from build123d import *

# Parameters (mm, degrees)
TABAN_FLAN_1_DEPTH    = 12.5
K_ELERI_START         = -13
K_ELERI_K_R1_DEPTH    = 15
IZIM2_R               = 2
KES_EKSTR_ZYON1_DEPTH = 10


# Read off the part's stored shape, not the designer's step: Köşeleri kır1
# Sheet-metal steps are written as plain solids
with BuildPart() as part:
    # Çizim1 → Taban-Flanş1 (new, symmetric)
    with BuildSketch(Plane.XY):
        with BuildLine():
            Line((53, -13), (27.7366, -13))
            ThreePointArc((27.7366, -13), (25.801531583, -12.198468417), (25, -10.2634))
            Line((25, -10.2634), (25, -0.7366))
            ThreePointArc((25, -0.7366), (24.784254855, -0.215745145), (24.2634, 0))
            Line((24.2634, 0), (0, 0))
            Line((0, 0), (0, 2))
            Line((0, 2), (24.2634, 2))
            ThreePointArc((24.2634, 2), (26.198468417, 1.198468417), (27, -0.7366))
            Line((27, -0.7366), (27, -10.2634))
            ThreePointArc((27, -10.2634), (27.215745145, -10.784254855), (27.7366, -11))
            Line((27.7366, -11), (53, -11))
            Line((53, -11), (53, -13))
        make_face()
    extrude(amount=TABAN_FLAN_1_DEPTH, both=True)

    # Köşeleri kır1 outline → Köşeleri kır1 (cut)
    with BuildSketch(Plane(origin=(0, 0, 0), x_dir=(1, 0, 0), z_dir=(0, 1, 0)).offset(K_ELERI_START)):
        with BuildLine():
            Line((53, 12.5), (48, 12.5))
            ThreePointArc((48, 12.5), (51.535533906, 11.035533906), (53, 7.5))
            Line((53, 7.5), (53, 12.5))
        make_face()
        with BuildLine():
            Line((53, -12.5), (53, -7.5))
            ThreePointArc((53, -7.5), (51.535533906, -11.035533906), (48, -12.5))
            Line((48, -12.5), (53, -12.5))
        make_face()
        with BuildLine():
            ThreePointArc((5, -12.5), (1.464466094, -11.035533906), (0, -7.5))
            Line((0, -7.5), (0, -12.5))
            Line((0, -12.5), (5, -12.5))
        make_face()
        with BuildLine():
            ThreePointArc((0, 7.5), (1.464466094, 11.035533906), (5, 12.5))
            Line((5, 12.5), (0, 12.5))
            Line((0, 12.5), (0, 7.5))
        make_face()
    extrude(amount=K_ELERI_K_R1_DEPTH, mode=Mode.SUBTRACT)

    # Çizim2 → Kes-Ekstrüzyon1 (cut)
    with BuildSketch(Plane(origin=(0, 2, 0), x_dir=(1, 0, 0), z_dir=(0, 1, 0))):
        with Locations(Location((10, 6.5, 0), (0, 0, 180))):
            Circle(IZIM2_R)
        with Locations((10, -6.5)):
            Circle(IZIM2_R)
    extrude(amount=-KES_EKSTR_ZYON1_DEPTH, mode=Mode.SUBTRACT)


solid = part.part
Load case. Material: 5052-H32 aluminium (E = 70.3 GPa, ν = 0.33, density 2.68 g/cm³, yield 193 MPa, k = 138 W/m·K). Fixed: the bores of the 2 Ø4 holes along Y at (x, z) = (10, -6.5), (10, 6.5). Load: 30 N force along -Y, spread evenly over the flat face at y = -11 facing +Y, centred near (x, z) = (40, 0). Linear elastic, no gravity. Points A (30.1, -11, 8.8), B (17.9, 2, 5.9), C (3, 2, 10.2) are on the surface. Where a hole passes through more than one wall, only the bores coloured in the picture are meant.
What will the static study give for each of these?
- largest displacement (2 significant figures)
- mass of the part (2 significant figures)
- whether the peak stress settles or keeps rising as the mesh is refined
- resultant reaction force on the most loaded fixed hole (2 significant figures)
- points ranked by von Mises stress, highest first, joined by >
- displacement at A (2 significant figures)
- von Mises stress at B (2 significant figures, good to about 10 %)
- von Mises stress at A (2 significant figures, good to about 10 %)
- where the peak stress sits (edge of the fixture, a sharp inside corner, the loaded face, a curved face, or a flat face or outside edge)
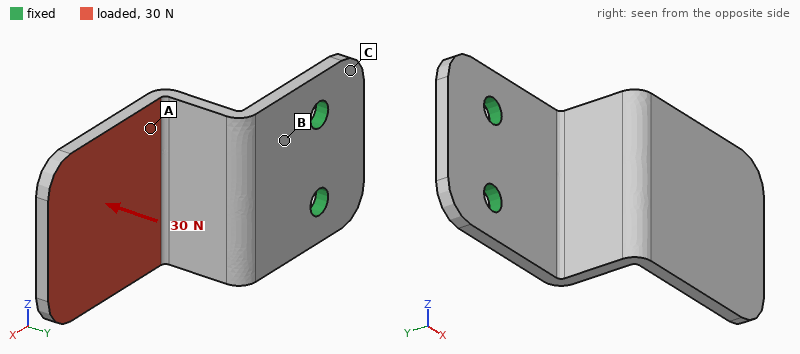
0.46 mm
8.4 g
keeps rising
15 N
B > A > C
0.16 mm
35 MPa
17 MPa
edge of the fixture
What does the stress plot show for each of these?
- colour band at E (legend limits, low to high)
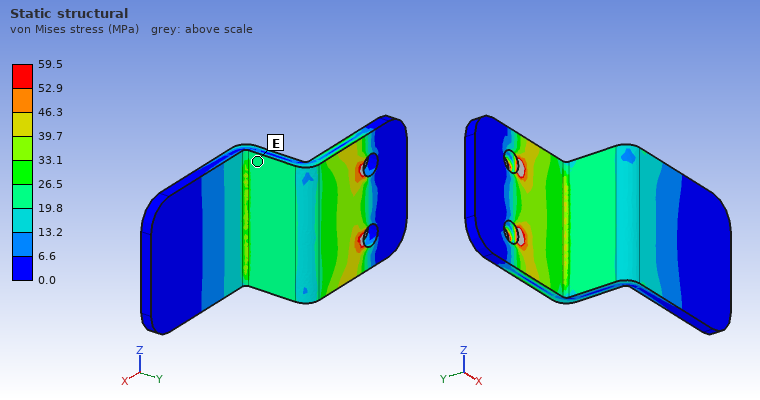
19.8 to 26.5 MPa
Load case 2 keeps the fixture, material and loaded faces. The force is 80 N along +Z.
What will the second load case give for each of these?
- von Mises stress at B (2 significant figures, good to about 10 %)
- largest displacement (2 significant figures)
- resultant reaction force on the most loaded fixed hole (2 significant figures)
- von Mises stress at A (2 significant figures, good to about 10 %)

18 MPa
0.14 mm
170 N
25 MPa
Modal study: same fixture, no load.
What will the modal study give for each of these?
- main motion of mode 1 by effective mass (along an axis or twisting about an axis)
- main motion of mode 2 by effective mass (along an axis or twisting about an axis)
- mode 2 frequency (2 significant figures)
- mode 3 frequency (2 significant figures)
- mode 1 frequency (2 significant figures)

along Y
along Z
2300 Hz
3000 Hz
770 Hz
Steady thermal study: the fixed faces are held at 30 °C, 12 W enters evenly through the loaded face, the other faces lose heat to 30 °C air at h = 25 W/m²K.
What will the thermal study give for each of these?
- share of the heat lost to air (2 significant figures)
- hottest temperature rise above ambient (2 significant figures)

16 %
62 K
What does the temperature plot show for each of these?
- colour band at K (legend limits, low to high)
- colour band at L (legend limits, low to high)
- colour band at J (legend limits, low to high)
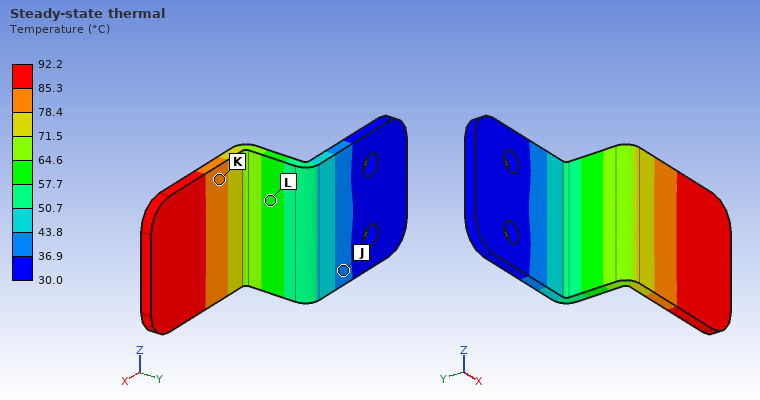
78.4 to 85.3 °C
57.7 to 64.6 °C
36.9 to 43.8 °C
